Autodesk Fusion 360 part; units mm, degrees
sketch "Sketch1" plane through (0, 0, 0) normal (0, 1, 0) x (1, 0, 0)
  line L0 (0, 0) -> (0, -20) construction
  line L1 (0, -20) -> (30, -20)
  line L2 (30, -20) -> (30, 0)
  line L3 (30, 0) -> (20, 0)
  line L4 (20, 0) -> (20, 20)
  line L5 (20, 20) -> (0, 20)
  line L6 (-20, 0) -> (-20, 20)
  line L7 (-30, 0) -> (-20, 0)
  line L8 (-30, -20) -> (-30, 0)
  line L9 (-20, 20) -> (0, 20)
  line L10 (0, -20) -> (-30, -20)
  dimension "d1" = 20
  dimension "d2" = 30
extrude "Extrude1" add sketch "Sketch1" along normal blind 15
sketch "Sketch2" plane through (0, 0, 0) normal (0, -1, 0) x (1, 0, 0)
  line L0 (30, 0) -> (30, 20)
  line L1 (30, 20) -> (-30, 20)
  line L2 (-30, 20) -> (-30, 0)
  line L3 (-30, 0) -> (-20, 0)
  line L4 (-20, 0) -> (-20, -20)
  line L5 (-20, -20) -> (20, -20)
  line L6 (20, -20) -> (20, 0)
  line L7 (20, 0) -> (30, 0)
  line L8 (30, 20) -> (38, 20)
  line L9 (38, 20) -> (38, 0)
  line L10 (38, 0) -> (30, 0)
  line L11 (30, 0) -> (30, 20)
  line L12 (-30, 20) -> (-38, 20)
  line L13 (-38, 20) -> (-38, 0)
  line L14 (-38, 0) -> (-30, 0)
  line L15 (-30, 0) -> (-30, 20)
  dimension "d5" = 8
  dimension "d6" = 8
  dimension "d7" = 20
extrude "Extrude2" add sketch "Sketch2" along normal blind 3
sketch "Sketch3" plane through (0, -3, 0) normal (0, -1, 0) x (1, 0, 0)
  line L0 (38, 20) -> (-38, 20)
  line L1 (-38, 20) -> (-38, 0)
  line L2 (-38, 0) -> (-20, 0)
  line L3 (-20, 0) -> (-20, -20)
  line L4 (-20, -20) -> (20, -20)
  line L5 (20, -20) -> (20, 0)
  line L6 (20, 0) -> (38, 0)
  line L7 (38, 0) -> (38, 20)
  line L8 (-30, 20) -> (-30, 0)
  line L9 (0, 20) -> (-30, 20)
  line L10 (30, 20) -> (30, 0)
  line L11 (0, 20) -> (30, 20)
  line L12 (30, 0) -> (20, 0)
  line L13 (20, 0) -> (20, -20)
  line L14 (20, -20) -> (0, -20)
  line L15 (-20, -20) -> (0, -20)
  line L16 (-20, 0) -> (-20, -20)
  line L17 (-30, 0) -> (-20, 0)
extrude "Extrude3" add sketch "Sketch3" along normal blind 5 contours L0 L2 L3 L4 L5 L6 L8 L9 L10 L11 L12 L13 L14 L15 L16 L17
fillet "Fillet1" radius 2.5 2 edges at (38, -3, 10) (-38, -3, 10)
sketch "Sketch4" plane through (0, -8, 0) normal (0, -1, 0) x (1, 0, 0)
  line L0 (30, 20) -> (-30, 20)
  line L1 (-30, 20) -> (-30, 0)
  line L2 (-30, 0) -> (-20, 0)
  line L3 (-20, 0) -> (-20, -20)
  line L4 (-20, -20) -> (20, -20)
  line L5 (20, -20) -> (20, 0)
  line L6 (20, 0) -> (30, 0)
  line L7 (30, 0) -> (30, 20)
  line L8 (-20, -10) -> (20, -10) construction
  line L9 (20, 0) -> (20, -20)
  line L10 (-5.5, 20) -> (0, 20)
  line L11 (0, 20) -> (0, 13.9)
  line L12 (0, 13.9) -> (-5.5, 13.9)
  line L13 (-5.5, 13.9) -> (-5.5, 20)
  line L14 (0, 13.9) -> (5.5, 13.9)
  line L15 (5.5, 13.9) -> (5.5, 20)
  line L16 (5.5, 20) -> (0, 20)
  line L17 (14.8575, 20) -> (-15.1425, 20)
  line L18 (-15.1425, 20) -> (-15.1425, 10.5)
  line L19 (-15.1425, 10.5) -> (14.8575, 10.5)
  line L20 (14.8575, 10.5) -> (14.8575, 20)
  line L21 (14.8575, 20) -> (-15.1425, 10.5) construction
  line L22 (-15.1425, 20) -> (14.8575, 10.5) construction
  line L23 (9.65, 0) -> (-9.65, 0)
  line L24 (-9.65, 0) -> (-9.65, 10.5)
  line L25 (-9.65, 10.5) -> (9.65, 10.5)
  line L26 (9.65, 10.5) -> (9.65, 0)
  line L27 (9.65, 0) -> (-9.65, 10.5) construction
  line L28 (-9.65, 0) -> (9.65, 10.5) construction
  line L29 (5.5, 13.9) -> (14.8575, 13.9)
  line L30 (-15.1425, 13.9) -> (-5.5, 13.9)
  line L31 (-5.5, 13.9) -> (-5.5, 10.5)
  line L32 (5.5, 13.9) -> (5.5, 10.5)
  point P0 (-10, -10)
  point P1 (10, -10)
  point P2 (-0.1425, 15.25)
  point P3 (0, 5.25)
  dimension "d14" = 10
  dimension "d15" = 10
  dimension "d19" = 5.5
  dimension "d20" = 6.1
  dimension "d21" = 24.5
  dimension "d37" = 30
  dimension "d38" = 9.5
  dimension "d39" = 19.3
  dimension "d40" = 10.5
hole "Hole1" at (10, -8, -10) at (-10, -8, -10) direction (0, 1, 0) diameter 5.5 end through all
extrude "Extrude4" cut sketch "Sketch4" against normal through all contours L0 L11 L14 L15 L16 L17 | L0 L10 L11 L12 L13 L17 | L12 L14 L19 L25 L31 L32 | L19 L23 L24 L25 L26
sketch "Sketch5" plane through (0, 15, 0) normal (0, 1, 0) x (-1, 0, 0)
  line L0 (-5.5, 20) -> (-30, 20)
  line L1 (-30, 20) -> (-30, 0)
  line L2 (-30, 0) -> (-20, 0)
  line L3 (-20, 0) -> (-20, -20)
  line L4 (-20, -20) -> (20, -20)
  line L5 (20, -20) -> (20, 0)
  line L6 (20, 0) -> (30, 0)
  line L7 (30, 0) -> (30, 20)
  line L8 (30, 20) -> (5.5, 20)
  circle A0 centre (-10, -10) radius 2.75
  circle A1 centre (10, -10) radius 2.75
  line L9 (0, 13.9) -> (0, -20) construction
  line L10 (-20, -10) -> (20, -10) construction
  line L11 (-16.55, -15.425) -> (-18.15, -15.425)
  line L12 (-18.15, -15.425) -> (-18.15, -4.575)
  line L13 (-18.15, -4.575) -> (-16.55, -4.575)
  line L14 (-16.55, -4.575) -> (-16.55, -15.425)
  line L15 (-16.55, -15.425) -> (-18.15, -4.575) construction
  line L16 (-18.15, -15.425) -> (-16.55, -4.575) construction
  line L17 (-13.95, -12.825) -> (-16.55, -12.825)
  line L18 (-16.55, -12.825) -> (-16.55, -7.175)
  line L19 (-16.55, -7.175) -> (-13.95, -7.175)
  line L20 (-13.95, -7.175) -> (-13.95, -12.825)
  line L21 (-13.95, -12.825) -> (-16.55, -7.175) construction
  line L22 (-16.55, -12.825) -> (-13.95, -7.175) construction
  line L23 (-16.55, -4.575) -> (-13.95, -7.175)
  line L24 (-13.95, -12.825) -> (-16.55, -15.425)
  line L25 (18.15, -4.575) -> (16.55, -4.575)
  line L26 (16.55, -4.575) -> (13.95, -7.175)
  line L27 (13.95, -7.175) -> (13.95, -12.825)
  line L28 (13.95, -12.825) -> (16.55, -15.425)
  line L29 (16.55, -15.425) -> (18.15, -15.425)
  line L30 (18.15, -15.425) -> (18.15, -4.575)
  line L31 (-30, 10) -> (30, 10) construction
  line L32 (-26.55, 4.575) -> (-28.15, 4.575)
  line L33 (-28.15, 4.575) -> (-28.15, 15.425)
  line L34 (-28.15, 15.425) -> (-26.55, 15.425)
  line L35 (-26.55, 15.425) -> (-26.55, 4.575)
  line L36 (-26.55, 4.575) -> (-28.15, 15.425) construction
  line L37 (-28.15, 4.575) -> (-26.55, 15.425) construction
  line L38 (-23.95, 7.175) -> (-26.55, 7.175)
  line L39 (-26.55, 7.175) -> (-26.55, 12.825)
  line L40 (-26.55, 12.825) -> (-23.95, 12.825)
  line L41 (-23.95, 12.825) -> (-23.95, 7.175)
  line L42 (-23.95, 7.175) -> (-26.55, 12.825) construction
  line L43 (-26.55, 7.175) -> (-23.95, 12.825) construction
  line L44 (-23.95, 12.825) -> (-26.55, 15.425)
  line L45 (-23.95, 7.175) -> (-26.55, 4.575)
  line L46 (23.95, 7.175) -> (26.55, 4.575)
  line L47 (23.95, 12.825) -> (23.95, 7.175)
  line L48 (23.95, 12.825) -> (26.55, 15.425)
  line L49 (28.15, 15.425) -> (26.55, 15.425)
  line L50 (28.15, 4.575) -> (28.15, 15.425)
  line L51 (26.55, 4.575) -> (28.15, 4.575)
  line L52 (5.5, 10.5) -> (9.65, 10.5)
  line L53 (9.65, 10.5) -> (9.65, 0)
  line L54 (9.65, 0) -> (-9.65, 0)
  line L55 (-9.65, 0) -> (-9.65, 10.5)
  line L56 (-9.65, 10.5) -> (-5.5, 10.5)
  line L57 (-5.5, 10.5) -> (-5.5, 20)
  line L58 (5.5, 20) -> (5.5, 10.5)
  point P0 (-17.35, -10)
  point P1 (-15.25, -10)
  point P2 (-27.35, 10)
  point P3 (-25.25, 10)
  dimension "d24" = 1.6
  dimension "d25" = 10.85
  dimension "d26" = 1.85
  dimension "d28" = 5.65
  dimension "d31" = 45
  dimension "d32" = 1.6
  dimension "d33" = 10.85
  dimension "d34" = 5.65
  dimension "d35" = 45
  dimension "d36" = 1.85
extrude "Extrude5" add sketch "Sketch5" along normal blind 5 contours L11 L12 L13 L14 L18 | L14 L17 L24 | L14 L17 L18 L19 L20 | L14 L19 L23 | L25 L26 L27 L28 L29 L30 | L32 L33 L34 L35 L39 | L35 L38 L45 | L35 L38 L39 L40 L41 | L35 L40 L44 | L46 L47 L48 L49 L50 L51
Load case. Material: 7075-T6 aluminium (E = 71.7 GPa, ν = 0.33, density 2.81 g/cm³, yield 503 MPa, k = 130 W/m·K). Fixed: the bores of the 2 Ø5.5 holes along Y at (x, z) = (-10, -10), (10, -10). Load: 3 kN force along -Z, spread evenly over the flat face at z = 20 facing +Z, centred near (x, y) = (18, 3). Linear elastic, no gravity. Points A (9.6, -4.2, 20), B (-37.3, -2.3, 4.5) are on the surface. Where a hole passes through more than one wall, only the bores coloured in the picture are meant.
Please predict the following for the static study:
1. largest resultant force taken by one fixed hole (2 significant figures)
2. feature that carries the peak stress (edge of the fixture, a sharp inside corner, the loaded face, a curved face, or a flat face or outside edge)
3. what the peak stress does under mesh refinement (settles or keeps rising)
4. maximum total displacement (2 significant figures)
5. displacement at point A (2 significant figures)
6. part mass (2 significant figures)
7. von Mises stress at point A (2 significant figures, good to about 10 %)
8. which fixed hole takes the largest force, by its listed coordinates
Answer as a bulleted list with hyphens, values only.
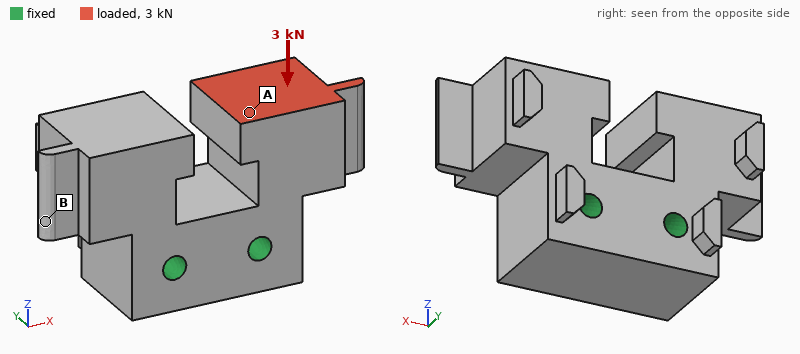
- 3.7 kN
- edge of the fixture
- keeps rising
- 35 µm
- 21 µm
- 110 g
- 6.3 MPa
- (10, -10)
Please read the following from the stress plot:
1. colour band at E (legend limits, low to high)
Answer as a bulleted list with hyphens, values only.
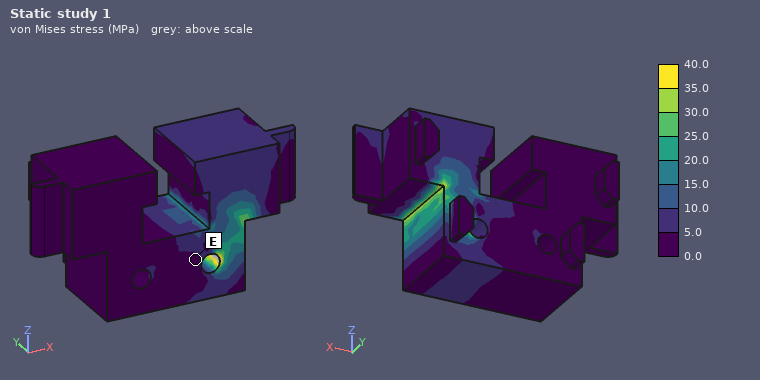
- 0.0 to 5.0 MPa
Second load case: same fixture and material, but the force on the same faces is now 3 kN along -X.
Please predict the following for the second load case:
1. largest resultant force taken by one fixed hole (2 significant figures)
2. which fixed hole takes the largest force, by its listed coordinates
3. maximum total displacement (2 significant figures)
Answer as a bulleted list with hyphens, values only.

- 3.3 kN
- (-10, -10)
- 0.15 mm
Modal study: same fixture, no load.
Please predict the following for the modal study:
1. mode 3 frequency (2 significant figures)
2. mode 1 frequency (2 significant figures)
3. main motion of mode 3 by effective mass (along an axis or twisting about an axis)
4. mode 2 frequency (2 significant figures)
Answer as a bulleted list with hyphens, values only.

- 11 kHz
- 6500 Hz
- twisting about Z
- 6600 Hz
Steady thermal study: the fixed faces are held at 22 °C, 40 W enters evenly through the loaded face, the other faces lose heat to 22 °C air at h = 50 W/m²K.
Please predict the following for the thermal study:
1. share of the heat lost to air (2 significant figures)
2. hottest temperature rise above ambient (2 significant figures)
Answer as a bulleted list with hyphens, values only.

- 6.5 %
- 24 K
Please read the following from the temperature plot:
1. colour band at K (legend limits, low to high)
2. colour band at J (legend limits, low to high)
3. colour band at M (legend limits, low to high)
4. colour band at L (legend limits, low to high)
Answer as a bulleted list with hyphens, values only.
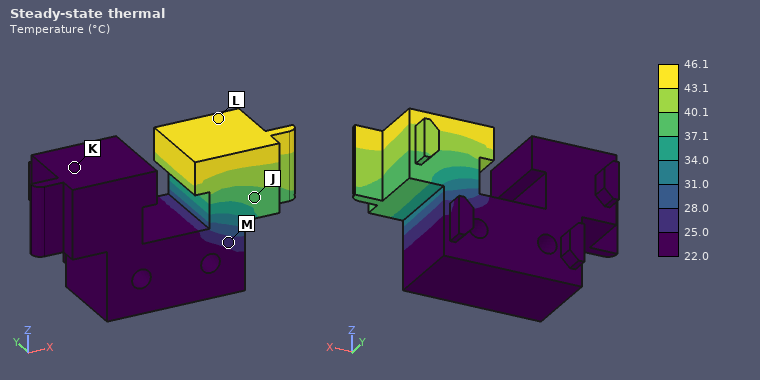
- 22.0 to 25.0 °C
- 37.1 to 40.1 °C
- 25.0 to 28.0 °C
- 43.1 to 46.1 °C
